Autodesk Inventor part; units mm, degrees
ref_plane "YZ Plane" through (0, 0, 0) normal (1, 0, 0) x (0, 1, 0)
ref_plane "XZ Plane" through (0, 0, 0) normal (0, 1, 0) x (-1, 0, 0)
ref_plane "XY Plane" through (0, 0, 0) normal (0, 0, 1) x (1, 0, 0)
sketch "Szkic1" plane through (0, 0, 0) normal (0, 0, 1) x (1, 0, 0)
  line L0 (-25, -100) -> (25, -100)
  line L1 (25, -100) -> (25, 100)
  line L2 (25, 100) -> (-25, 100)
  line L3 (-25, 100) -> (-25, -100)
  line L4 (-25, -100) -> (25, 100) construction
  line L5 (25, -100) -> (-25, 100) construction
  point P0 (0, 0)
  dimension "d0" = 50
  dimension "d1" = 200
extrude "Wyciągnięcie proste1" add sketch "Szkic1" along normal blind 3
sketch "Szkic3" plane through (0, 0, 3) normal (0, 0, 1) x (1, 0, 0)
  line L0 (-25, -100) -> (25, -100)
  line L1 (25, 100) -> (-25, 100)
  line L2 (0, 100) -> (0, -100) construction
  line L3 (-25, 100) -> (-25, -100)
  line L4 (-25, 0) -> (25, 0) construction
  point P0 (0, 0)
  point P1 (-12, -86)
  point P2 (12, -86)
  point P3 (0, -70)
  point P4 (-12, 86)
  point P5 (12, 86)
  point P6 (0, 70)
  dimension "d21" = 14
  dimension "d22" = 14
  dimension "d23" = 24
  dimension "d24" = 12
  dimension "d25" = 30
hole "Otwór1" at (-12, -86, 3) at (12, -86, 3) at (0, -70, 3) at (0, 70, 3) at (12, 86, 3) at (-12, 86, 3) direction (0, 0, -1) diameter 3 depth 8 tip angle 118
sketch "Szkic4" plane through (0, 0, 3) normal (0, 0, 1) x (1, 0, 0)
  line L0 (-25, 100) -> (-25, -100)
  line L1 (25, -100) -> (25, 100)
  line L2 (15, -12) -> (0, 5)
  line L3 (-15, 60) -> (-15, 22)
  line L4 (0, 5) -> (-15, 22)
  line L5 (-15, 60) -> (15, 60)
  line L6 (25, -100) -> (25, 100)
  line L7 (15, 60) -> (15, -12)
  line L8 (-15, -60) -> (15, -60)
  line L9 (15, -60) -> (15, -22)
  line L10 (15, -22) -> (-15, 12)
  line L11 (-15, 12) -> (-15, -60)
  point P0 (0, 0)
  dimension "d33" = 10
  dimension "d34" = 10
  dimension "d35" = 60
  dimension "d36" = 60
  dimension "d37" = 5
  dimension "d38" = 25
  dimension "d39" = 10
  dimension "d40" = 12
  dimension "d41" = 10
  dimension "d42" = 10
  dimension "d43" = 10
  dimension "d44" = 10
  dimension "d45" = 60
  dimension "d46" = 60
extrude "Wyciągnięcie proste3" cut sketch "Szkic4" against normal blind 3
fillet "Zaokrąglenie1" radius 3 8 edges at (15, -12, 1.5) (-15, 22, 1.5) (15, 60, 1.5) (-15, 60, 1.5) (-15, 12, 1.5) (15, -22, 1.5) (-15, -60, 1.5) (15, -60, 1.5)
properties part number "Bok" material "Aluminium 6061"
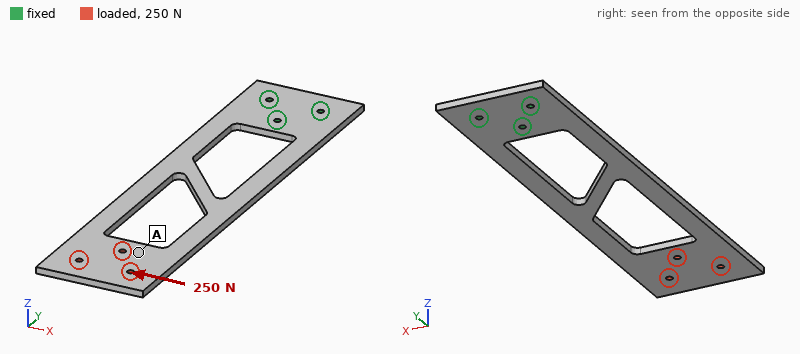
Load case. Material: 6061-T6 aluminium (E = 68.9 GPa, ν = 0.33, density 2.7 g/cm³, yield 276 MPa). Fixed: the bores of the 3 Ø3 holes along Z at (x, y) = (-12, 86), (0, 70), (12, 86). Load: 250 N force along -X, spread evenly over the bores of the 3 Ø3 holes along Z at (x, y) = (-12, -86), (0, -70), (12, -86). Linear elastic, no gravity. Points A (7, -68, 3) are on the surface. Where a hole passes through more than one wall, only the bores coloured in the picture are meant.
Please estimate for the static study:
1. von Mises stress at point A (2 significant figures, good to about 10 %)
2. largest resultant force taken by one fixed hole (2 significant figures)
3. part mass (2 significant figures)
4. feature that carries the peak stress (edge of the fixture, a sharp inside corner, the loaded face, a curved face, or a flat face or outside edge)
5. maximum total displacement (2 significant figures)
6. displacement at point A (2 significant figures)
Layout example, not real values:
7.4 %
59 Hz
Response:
14 MPa
1.1 kN
54 g
a curved face
0.62 mm
0.55 mm
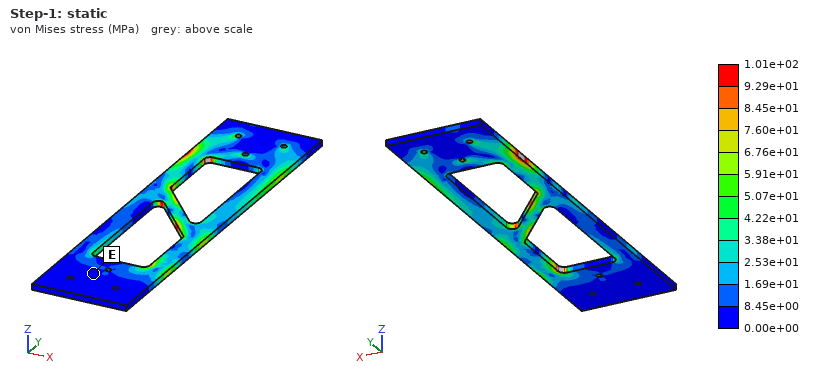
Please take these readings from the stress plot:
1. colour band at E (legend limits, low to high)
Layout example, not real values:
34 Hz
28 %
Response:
0.00e+00 to 8.45e+00 MPa
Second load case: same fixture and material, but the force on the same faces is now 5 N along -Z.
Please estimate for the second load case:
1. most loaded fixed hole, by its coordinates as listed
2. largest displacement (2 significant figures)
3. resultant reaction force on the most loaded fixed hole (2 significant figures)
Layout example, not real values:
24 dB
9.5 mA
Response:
(0, 70)
2.1 mm
36 N
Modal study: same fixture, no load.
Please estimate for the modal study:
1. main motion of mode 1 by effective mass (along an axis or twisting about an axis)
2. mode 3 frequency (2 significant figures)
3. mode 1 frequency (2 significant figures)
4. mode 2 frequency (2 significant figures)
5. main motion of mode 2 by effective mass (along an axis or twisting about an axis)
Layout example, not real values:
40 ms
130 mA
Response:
along Z
450 Hz
62 Hz
370 Hz
twisting about Y
